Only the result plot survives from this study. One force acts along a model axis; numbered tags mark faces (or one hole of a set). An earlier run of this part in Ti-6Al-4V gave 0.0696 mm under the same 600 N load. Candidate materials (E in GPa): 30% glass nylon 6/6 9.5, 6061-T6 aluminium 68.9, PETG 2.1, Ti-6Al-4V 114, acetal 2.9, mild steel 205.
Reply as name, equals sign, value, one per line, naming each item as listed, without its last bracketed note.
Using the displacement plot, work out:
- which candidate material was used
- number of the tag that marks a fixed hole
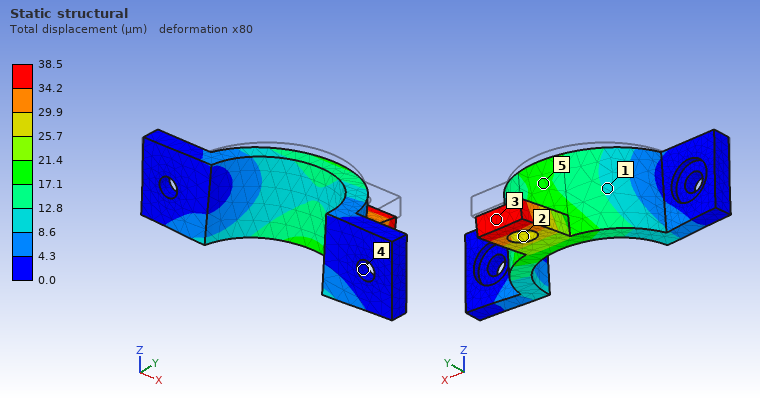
which candidate material was used = mild steel
number of the tag that marks a fixed hole = 4
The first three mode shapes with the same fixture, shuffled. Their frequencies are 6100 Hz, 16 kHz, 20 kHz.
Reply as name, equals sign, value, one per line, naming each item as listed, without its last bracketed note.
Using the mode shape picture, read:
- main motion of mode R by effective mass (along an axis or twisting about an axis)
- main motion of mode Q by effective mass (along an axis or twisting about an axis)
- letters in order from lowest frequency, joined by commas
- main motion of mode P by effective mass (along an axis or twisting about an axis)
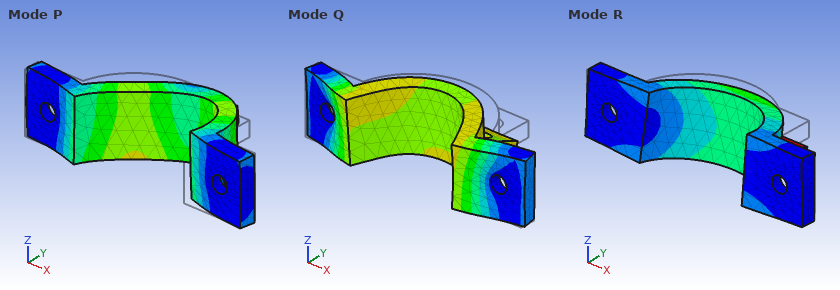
main motion of mode R by effective mass = along Z
main motion of mode Q by effective mass = along Y
letters in order from lowest frequency, joined by commas = R, P, Q
main motion of mode P by effective mass = along X
